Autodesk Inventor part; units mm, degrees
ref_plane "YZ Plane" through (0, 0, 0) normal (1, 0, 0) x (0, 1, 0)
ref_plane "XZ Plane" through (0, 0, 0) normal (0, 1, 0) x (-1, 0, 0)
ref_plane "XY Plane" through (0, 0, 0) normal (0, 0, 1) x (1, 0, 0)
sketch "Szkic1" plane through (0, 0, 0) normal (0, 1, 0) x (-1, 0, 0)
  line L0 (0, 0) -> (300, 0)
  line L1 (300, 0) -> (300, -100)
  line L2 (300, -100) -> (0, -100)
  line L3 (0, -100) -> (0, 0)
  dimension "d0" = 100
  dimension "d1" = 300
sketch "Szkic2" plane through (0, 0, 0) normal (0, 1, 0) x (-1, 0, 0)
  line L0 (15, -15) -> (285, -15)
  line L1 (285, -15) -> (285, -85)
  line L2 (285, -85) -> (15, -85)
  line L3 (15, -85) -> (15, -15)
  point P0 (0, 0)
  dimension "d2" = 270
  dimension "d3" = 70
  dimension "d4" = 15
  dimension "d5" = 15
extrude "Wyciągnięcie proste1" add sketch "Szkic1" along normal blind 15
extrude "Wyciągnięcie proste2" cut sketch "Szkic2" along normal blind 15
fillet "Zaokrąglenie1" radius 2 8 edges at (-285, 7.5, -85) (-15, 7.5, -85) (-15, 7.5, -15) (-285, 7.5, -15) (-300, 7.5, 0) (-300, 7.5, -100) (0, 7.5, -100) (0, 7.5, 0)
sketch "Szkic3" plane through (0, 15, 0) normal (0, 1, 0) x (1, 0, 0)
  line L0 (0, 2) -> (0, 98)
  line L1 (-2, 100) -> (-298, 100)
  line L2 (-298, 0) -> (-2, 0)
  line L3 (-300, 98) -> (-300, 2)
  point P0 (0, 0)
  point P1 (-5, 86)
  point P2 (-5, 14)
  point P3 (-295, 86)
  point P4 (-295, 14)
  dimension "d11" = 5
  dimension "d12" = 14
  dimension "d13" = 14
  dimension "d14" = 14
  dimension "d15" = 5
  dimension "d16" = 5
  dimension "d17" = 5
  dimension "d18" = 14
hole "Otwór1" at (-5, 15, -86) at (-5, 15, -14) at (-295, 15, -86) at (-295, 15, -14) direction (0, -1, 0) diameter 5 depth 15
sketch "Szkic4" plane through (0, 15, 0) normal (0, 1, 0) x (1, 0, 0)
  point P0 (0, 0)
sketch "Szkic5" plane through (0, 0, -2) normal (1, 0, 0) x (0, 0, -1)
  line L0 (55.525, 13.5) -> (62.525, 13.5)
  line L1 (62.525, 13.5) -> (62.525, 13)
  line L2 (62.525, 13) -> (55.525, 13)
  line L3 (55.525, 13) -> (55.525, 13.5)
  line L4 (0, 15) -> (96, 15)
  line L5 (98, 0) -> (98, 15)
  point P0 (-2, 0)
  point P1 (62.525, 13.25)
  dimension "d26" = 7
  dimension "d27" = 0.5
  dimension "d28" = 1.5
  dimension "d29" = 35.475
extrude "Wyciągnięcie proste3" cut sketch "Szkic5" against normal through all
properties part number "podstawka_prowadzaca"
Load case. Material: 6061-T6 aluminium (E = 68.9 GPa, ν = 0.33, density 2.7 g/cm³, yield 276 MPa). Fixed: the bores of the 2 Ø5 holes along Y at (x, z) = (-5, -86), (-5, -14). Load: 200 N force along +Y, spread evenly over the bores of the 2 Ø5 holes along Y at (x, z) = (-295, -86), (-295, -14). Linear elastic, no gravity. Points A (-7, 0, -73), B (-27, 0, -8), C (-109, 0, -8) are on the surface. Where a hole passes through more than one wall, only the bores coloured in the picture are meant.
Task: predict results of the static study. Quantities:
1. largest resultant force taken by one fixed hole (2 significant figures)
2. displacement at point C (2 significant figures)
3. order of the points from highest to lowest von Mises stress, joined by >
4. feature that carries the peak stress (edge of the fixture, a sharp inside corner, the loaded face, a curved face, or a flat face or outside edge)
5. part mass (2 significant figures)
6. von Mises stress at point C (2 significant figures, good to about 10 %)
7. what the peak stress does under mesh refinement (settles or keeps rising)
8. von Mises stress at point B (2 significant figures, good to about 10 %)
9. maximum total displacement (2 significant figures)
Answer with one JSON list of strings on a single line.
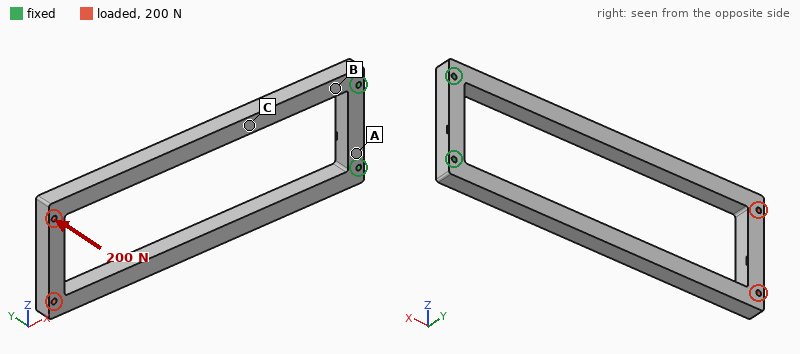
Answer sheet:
["100 N", "0.50 mm", "B > C > A", "edge of the fixture", "450 g", "33 MPa", "keeps rising", "48 MPa", "2.9 mm"]
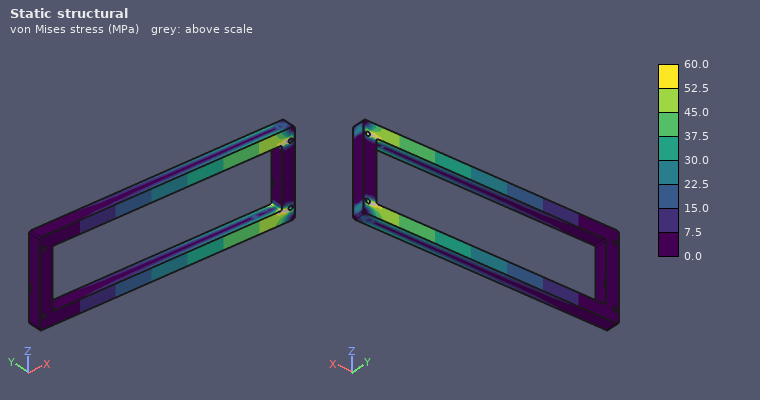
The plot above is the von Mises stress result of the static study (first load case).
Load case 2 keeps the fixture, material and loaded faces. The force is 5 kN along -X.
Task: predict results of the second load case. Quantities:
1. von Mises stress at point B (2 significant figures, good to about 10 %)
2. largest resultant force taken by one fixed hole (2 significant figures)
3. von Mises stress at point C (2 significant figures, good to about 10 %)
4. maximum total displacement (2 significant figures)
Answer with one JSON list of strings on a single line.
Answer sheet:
["11 MPa", "2.5 kN", "11 MPa", "92 µm"]
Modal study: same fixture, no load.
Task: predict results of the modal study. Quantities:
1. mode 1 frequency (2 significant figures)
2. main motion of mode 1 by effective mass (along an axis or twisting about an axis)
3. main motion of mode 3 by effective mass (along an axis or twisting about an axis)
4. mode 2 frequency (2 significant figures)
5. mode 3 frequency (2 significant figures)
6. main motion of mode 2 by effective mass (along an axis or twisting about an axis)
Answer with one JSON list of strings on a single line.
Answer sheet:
["120 Hz", "along Y", "twisting about X", "190 Hz", "400 Hz", "along Z"]
